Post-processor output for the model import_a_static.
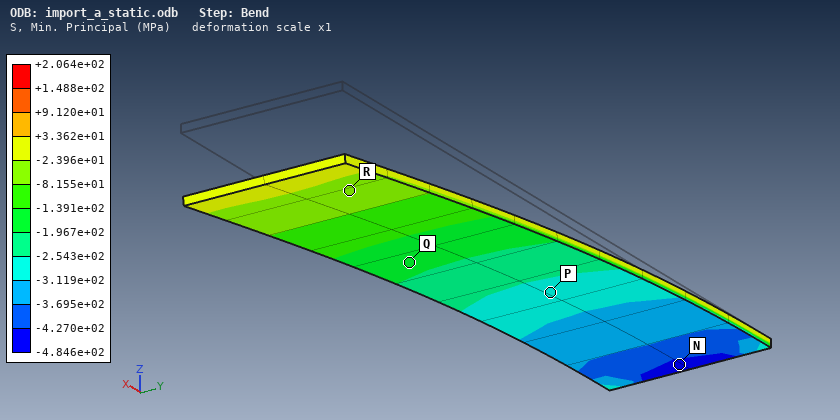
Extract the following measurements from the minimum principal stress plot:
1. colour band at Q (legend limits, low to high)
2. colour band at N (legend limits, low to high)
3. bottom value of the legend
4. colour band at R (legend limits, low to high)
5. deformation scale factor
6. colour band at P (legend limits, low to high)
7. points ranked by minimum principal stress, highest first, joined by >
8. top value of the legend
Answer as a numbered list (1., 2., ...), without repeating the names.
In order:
1. -1.967e+02 to -1.391e+02 MPa
2. -4.846e+02 to -4.270e+02 MPa
3. -4.846e+02 MPa
4. -8.155e+01 to -2.396e+01 MPa
5. 1
6. -3.119e+02 to -2.543e+02 MPa
7. R > Q > P > N
8. +2.064e+02 MPa
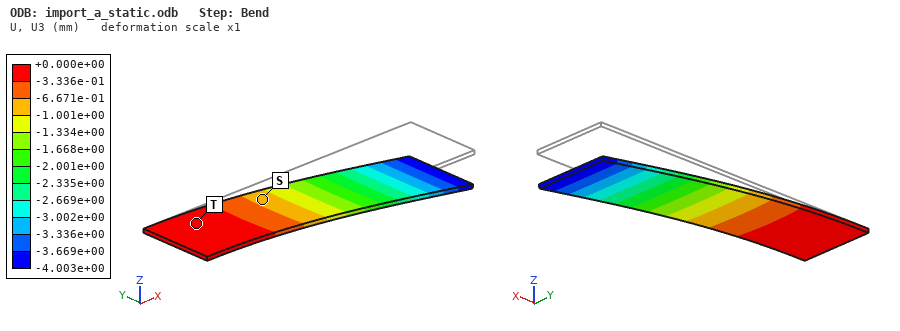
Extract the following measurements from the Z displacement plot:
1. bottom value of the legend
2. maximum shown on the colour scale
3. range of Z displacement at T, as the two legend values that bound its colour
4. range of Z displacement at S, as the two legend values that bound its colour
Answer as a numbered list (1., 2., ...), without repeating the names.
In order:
1. -4.003e+00 mm
2. +0.000e+00 mm
3. -3.336e-01 to +0.000e+00 mm
4. -1.001e+00 to -6.671e-01 mm
